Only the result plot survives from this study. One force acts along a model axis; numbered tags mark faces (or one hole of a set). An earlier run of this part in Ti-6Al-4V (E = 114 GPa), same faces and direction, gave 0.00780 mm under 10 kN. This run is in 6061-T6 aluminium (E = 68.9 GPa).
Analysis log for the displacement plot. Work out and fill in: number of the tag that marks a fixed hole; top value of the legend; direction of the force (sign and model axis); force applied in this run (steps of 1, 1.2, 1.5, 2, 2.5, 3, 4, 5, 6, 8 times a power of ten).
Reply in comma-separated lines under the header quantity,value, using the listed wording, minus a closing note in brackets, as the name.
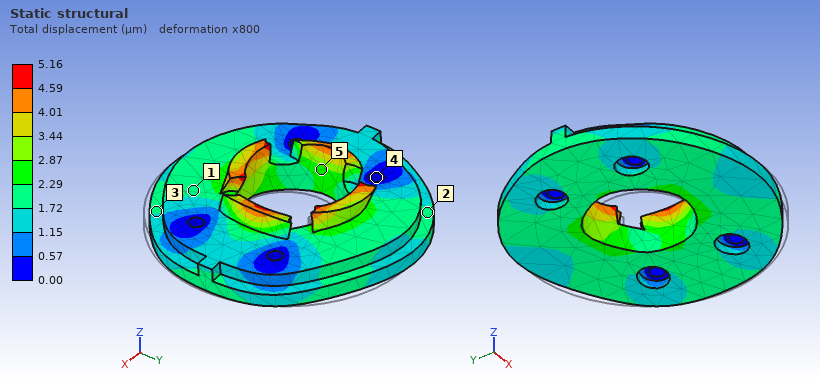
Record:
quantity,value
number of the tag that marks a fixed hole,4
top value of the legend,5.16 µm
direction of the force,-X
force applied in this run,4 kN
